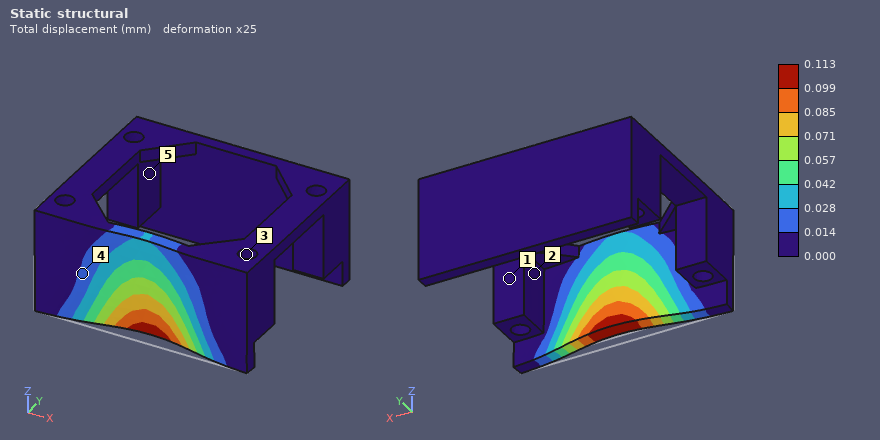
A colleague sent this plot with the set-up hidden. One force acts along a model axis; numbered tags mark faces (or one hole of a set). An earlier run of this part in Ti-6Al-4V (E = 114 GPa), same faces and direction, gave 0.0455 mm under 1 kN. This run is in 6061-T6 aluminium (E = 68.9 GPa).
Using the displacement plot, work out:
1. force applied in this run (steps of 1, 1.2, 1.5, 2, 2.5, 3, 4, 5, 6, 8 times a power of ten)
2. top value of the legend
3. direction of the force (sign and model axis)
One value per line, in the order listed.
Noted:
1.5 kN
0.113 mm
+Y
